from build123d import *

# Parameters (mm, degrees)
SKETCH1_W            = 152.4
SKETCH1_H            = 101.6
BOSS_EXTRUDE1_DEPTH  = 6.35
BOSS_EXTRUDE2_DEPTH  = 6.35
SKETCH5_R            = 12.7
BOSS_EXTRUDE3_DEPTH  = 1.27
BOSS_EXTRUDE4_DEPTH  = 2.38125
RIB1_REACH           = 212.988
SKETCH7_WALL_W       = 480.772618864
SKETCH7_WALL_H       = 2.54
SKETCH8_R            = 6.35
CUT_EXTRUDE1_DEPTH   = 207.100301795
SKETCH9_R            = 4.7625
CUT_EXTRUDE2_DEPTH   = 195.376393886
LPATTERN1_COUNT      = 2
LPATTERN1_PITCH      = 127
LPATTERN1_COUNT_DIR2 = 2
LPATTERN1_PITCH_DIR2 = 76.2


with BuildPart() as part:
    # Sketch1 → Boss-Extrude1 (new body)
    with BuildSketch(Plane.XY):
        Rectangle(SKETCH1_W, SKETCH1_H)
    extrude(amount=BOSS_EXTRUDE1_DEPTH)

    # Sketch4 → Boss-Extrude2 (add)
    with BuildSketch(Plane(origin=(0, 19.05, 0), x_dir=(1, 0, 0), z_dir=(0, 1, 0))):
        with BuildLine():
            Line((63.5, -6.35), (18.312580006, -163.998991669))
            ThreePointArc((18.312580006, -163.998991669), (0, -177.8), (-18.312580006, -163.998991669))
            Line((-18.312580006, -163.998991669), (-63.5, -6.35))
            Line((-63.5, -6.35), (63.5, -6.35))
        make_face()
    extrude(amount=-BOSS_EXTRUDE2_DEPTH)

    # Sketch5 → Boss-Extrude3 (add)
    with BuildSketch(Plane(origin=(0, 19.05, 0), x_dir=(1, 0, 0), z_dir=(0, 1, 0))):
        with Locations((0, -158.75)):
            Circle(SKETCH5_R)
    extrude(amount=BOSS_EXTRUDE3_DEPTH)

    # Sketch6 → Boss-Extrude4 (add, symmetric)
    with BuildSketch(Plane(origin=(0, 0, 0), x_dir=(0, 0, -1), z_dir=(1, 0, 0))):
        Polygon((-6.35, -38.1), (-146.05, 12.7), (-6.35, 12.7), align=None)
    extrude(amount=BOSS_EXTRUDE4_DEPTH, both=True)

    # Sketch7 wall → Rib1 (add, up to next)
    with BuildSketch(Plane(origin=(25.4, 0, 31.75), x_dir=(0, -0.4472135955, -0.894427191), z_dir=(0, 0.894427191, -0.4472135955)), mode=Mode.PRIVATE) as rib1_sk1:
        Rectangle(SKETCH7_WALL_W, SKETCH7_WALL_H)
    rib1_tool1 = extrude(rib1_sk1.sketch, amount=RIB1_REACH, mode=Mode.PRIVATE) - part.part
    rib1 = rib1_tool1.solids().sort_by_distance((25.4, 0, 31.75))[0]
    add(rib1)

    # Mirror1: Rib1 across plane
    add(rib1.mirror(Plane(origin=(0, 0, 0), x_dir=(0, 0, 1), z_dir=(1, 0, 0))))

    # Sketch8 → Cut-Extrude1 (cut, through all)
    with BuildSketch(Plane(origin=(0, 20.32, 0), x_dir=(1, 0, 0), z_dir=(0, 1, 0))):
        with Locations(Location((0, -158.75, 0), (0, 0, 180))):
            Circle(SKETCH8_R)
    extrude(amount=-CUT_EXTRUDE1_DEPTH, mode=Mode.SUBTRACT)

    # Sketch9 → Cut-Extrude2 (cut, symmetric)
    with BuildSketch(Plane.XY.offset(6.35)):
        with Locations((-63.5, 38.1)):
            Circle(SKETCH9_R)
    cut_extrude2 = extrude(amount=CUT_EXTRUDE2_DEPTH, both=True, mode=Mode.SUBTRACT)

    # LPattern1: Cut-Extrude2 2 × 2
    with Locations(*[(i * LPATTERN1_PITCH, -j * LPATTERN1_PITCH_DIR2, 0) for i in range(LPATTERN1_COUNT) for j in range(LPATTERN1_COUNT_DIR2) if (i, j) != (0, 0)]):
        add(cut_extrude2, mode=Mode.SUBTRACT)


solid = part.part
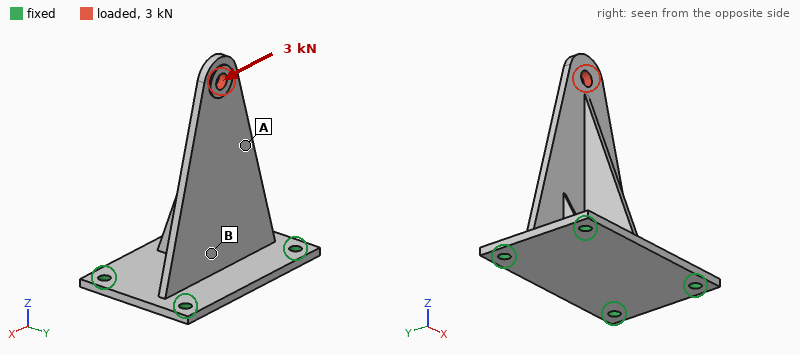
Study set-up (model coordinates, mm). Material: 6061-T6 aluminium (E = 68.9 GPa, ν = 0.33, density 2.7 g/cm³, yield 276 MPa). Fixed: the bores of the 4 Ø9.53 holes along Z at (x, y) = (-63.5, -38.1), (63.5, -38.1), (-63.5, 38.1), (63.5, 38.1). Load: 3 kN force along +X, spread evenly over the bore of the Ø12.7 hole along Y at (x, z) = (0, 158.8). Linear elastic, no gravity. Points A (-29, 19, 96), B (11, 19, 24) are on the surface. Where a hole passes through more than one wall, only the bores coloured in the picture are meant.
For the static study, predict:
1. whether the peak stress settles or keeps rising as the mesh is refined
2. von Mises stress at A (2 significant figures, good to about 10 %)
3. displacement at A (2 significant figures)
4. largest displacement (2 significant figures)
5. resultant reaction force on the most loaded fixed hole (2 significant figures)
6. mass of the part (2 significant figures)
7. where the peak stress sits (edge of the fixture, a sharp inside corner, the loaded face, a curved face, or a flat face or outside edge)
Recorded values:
keeps rising
27 MPa
0.19 mm
0.41 mm
3.3 kN
540 g
edge of the fixture
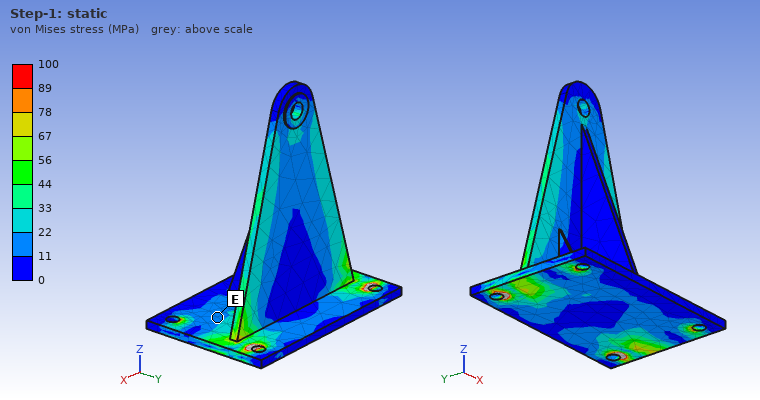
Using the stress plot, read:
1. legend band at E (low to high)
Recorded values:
11 to 22 MPa
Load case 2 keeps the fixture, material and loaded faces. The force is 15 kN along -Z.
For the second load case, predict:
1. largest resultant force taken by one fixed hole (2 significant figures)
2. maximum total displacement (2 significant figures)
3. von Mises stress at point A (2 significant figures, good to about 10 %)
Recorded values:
6.2 kN
0.63 mm
39 MPa
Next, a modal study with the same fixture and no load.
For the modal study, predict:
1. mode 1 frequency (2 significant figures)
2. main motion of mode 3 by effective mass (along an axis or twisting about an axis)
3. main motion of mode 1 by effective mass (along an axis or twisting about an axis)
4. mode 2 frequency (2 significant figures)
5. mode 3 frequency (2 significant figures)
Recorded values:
580 Hz
along X
along Y
1500 Hz
1800 Hz
